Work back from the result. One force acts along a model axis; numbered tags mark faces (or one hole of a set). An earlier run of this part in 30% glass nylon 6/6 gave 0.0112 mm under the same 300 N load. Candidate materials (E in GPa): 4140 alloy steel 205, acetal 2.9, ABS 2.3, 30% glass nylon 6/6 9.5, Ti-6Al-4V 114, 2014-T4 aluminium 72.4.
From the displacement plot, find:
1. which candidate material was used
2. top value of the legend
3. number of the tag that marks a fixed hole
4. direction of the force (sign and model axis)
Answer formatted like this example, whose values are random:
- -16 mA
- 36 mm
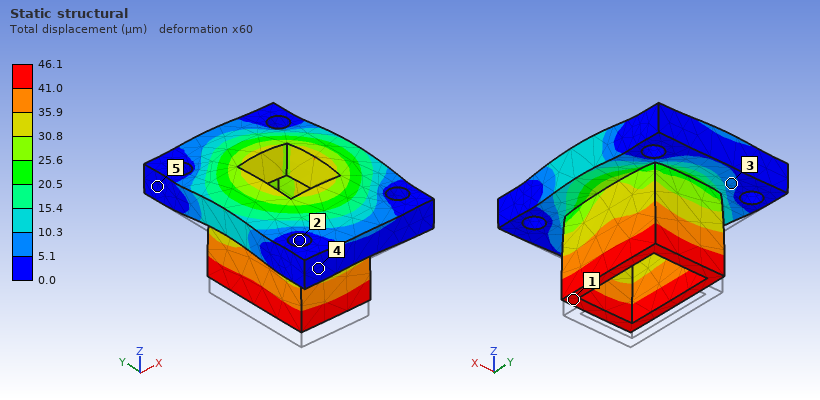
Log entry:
- ABS
- 46.1 µm
- 2
- +Z
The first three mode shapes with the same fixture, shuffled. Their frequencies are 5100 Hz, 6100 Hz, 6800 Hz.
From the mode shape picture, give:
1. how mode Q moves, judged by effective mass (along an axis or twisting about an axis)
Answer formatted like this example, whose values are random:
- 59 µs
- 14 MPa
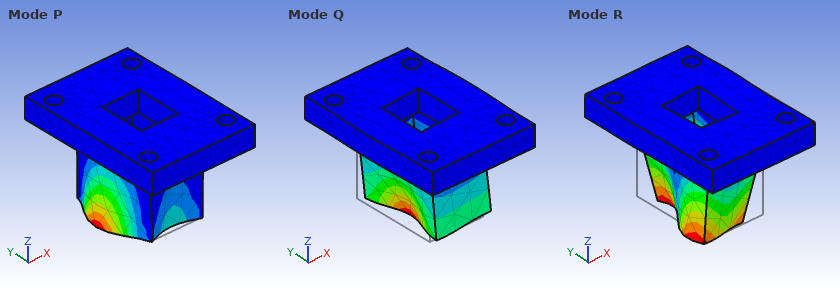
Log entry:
- along X
